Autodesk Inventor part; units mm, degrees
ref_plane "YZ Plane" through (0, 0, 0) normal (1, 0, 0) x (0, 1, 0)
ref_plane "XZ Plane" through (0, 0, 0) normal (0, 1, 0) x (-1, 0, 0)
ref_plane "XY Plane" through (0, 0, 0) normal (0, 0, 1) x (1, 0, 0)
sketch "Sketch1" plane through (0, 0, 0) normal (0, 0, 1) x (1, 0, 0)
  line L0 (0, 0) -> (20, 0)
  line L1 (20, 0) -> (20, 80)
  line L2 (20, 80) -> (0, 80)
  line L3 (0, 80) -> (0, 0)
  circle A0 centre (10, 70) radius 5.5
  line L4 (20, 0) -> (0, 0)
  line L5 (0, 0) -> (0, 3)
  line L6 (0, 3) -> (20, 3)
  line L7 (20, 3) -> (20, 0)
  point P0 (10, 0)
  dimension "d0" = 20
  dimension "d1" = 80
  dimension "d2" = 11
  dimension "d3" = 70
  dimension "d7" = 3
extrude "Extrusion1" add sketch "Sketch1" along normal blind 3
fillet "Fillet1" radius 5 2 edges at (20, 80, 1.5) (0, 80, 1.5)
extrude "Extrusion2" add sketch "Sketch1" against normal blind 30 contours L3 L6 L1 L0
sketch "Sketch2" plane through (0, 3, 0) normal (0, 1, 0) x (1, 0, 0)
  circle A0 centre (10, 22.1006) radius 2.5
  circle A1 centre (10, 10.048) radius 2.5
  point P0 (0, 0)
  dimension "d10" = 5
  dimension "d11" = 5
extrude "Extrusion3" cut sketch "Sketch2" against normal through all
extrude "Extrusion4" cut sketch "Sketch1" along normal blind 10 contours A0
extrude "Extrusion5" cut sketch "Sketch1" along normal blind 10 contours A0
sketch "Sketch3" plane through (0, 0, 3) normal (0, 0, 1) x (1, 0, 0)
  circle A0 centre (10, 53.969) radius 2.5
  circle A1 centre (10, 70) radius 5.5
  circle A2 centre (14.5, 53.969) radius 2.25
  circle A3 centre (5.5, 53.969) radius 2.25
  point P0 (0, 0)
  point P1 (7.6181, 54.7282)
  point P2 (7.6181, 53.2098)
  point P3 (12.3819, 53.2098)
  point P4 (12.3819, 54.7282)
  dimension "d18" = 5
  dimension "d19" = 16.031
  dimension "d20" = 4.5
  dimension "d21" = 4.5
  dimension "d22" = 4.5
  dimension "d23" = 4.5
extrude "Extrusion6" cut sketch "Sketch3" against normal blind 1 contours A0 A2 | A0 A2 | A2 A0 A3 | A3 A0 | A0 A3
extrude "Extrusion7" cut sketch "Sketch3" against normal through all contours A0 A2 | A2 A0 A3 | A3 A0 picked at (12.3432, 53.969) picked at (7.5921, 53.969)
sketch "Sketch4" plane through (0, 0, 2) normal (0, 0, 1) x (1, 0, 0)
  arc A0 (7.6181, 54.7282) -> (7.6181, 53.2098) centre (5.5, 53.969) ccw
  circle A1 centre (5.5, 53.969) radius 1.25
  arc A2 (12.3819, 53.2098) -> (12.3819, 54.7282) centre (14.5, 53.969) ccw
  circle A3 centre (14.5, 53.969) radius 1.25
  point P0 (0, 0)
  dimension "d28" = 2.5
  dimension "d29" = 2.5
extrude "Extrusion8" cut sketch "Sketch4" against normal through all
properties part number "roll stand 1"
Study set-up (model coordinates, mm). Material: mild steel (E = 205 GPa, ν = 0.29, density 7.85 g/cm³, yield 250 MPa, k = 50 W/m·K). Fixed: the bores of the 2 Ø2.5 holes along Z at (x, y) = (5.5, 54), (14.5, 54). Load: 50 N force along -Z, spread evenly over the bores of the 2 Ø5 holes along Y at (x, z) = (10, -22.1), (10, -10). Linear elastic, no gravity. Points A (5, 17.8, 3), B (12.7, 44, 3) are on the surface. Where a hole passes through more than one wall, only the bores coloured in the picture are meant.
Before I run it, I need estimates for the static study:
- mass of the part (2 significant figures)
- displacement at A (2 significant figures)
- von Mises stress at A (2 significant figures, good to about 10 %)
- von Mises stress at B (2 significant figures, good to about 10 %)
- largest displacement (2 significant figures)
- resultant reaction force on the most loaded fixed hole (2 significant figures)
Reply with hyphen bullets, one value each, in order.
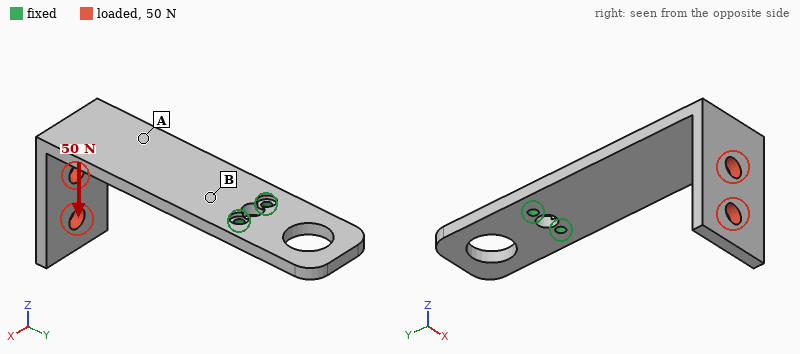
- 48 g
- 0.18 mm
- 27 MPa
- 65 MPa
- 0.42 mm
- 33 N
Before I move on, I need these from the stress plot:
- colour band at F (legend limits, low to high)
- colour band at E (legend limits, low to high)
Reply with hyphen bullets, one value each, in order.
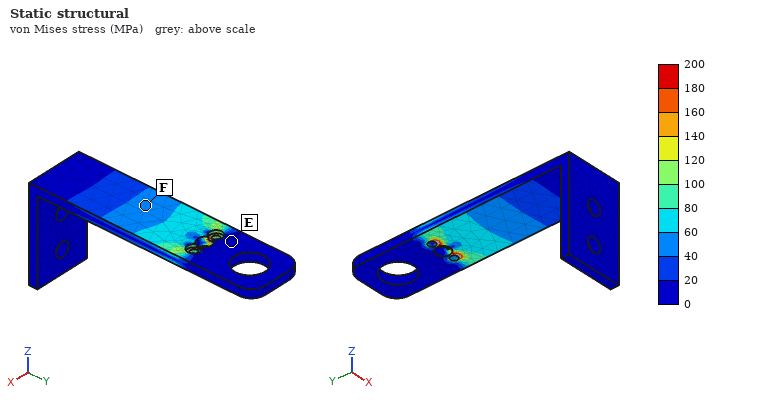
- 40 to 60 MPa
- 0 to 20 MPa
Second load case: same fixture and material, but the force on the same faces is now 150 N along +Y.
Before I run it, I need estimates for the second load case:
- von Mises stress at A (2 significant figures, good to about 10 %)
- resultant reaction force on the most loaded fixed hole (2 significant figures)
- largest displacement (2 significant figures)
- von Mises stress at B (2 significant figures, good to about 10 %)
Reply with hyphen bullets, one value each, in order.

- 84 MPa
- 75 N
- 0.74 mm
- 79 MPa
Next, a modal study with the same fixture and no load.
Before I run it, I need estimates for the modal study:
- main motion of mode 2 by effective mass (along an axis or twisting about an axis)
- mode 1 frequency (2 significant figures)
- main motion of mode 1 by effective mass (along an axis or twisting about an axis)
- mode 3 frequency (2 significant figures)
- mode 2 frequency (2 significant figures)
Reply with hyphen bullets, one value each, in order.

- along X
- 410 Hz
- along Z
- 1600 Hz
- 1100 Hz
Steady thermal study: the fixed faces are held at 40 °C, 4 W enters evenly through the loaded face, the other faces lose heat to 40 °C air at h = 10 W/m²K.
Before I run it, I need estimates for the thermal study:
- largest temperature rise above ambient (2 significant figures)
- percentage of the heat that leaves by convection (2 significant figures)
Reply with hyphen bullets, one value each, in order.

- 70 K
- 37 %
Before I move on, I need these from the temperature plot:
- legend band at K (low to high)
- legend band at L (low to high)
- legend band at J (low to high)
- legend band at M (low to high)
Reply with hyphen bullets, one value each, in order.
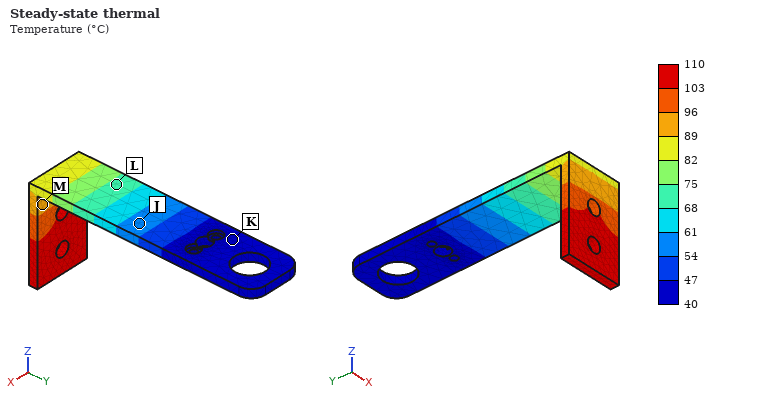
- 40 to 47 °C
- 68 to 75 °C
- 54 to 61 °C
- 89 to 96 °C
